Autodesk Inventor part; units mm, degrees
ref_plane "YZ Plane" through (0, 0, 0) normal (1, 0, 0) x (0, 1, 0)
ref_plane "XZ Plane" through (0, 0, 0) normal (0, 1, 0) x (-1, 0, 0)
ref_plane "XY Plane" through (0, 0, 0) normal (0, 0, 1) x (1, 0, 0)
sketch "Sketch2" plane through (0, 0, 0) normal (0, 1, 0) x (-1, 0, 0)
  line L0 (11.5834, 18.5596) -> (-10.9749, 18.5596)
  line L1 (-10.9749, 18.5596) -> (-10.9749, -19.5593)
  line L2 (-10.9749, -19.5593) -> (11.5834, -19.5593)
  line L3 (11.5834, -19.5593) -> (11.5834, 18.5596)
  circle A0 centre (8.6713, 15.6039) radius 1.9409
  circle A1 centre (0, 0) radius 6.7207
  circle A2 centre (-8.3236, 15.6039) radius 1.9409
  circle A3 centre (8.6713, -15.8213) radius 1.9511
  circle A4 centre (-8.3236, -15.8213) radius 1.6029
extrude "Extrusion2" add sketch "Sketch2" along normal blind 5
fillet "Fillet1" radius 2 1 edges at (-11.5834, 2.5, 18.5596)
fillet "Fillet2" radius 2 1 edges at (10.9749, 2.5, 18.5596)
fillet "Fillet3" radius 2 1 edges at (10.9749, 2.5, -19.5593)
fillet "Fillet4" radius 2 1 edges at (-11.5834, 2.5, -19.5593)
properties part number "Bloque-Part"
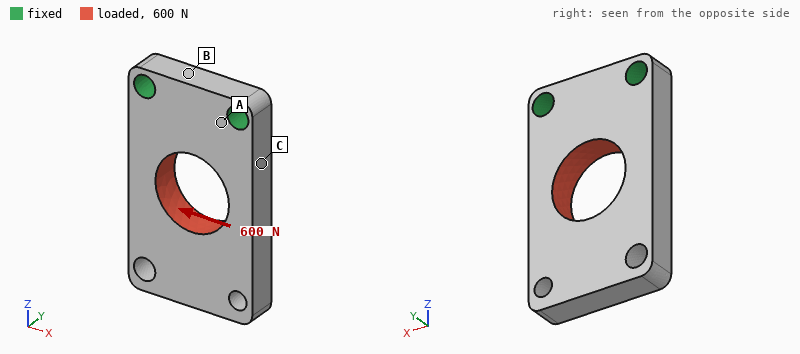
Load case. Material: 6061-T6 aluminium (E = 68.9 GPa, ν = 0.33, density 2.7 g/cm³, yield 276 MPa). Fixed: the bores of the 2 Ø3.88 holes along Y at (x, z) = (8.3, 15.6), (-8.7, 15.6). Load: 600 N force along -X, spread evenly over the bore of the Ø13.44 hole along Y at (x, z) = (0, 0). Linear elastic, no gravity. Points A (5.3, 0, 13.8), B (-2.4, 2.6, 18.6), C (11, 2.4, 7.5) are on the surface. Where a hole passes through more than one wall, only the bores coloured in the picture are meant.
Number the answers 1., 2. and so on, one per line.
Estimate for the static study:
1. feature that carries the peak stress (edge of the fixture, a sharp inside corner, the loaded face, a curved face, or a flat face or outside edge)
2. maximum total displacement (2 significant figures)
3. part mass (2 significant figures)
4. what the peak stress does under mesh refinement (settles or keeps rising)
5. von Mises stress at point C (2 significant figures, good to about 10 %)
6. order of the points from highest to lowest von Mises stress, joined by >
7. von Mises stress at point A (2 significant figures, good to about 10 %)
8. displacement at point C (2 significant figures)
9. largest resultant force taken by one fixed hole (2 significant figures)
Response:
1. edge of the fixture
2. 21 µm
3. 9.1 g
4. keeps rising
5. 28 MPa
6. C > A > B
7. 11 MPa
8. 4.1 µm
9. 570 N
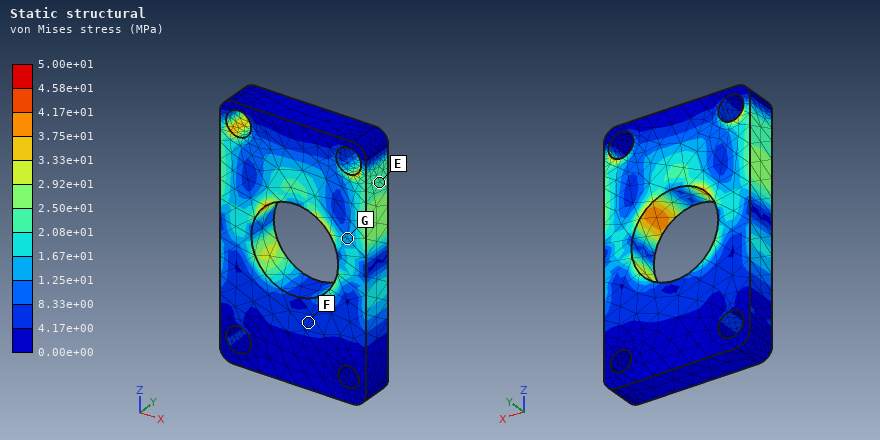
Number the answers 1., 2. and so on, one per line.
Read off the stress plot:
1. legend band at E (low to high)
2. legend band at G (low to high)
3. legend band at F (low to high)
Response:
1. 2.08e+01 to 2.50e+01 MPa
2. 1.25e+01 to 1.67e+01 MPa
3. 4.17e+00 to 8.33e+00 MPa
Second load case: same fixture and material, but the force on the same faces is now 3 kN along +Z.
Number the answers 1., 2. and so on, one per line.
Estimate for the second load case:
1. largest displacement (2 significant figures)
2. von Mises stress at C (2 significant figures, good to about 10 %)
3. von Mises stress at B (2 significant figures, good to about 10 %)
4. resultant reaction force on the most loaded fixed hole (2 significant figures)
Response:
1. 14 µm
2. 48 MPa
3. 12 MPa
4. 1.6 kN
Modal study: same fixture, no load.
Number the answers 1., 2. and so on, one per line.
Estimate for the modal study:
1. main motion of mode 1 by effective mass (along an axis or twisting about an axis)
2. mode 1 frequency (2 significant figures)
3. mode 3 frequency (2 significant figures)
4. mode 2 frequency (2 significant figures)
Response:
1. along Y
2. 3000 Hz
3. 9300 Hz
4. 9200 Hz
